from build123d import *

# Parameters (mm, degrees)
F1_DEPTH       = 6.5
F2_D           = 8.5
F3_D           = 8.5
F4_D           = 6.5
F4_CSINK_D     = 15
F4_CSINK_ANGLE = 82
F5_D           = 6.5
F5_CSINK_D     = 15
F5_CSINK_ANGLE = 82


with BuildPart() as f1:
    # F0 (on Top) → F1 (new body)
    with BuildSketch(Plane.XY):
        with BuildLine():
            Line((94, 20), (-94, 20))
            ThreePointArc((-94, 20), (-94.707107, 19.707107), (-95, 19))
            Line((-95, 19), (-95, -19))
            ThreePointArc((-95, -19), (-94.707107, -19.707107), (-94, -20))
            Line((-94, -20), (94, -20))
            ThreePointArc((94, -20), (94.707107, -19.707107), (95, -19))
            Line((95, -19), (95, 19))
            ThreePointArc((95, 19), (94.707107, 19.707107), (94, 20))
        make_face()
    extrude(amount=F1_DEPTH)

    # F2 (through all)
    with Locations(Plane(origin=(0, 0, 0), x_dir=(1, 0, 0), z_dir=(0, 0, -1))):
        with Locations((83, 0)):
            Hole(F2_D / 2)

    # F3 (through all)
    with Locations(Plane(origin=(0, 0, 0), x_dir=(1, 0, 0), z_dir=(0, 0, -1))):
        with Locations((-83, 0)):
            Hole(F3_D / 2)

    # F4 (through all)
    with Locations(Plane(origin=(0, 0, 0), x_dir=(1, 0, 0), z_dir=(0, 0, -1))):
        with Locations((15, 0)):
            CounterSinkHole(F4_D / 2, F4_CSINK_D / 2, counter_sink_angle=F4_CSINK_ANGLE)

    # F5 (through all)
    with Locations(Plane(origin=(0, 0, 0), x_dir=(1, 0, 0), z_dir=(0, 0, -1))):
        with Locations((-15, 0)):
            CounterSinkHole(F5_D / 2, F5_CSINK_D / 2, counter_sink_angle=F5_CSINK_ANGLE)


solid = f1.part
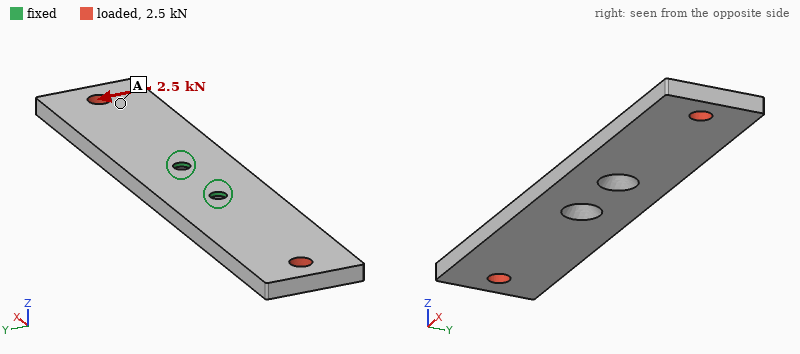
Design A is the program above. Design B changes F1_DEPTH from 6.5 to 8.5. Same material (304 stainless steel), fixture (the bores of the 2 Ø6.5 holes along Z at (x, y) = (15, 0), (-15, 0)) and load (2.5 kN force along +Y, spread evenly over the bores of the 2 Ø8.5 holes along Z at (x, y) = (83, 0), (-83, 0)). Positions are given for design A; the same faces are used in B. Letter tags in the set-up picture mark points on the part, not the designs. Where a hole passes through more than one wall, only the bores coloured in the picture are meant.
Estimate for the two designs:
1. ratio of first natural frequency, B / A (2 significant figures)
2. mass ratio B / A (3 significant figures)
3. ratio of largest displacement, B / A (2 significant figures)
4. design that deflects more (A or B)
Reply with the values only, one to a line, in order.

1.3
1.31
0.72
A
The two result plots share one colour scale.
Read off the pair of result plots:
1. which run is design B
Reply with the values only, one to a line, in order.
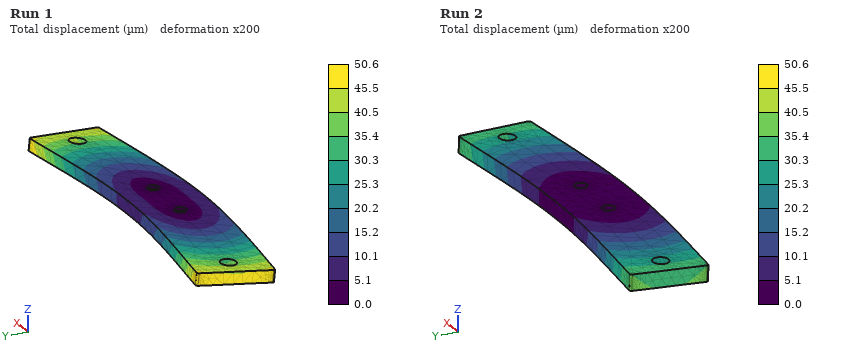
Run 2
